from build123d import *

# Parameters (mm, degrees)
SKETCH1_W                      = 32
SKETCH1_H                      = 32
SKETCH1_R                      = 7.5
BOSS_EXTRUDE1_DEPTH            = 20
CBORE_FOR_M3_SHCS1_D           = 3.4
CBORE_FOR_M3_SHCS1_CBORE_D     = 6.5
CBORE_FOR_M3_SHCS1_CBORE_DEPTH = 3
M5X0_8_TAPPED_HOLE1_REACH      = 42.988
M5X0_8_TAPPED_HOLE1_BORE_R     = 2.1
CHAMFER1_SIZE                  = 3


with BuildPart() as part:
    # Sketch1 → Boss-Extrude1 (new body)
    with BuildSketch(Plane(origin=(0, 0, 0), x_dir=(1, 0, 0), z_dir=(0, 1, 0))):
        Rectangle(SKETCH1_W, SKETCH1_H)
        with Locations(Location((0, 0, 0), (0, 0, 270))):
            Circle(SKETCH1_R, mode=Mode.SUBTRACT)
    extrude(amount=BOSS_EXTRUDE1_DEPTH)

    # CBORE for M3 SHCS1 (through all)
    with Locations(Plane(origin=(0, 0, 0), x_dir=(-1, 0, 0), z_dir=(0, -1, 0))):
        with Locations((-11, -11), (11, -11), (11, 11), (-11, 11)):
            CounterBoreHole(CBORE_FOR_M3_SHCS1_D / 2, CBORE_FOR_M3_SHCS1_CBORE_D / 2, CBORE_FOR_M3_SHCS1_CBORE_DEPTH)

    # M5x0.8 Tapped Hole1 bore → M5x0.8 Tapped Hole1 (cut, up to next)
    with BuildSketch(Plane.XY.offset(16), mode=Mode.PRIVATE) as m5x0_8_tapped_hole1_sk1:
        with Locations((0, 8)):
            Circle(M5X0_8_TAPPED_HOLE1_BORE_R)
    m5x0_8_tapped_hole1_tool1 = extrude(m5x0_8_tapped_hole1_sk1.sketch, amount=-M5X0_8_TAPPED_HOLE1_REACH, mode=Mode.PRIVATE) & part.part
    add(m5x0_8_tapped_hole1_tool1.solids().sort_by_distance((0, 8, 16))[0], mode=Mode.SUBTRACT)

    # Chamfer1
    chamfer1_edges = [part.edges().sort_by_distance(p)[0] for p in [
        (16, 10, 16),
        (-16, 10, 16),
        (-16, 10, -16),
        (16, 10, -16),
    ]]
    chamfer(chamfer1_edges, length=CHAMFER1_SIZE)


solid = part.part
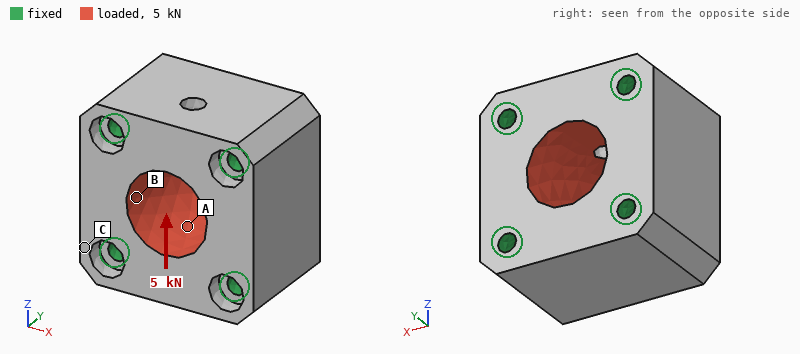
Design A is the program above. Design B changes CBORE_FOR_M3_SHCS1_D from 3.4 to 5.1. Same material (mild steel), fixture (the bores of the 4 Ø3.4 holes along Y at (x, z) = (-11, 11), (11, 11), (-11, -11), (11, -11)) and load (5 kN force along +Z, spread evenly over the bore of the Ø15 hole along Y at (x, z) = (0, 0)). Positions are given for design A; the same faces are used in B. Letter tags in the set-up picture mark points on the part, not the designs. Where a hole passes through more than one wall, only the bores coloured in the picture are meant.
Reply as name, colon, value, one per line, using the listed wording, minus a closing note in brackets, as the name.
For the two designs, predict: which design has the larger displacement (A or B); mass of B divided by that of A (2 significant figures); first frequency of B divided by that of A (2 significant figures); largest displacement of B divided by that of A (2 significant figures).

which design has the larger displacement: A
mass of B divided by that of A: 0.95
first frequency of B divided by that of A: 1.2
largest displacement of B divided by that of A: 0.86
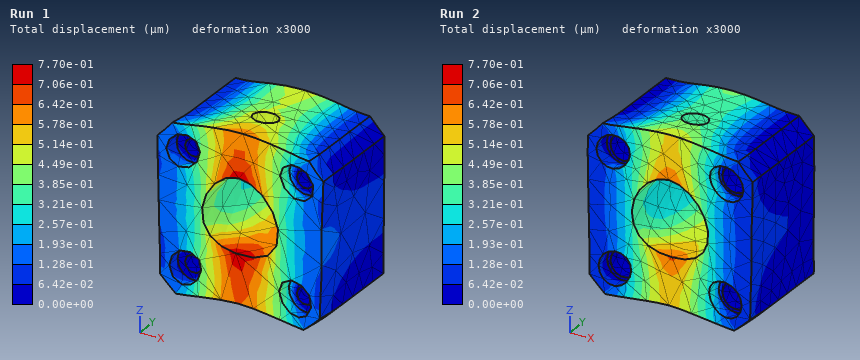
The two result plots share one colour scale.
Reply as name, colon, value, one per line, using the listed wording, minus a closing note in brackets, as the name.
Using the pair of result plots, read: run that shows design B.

run that shows design B: Run 2
